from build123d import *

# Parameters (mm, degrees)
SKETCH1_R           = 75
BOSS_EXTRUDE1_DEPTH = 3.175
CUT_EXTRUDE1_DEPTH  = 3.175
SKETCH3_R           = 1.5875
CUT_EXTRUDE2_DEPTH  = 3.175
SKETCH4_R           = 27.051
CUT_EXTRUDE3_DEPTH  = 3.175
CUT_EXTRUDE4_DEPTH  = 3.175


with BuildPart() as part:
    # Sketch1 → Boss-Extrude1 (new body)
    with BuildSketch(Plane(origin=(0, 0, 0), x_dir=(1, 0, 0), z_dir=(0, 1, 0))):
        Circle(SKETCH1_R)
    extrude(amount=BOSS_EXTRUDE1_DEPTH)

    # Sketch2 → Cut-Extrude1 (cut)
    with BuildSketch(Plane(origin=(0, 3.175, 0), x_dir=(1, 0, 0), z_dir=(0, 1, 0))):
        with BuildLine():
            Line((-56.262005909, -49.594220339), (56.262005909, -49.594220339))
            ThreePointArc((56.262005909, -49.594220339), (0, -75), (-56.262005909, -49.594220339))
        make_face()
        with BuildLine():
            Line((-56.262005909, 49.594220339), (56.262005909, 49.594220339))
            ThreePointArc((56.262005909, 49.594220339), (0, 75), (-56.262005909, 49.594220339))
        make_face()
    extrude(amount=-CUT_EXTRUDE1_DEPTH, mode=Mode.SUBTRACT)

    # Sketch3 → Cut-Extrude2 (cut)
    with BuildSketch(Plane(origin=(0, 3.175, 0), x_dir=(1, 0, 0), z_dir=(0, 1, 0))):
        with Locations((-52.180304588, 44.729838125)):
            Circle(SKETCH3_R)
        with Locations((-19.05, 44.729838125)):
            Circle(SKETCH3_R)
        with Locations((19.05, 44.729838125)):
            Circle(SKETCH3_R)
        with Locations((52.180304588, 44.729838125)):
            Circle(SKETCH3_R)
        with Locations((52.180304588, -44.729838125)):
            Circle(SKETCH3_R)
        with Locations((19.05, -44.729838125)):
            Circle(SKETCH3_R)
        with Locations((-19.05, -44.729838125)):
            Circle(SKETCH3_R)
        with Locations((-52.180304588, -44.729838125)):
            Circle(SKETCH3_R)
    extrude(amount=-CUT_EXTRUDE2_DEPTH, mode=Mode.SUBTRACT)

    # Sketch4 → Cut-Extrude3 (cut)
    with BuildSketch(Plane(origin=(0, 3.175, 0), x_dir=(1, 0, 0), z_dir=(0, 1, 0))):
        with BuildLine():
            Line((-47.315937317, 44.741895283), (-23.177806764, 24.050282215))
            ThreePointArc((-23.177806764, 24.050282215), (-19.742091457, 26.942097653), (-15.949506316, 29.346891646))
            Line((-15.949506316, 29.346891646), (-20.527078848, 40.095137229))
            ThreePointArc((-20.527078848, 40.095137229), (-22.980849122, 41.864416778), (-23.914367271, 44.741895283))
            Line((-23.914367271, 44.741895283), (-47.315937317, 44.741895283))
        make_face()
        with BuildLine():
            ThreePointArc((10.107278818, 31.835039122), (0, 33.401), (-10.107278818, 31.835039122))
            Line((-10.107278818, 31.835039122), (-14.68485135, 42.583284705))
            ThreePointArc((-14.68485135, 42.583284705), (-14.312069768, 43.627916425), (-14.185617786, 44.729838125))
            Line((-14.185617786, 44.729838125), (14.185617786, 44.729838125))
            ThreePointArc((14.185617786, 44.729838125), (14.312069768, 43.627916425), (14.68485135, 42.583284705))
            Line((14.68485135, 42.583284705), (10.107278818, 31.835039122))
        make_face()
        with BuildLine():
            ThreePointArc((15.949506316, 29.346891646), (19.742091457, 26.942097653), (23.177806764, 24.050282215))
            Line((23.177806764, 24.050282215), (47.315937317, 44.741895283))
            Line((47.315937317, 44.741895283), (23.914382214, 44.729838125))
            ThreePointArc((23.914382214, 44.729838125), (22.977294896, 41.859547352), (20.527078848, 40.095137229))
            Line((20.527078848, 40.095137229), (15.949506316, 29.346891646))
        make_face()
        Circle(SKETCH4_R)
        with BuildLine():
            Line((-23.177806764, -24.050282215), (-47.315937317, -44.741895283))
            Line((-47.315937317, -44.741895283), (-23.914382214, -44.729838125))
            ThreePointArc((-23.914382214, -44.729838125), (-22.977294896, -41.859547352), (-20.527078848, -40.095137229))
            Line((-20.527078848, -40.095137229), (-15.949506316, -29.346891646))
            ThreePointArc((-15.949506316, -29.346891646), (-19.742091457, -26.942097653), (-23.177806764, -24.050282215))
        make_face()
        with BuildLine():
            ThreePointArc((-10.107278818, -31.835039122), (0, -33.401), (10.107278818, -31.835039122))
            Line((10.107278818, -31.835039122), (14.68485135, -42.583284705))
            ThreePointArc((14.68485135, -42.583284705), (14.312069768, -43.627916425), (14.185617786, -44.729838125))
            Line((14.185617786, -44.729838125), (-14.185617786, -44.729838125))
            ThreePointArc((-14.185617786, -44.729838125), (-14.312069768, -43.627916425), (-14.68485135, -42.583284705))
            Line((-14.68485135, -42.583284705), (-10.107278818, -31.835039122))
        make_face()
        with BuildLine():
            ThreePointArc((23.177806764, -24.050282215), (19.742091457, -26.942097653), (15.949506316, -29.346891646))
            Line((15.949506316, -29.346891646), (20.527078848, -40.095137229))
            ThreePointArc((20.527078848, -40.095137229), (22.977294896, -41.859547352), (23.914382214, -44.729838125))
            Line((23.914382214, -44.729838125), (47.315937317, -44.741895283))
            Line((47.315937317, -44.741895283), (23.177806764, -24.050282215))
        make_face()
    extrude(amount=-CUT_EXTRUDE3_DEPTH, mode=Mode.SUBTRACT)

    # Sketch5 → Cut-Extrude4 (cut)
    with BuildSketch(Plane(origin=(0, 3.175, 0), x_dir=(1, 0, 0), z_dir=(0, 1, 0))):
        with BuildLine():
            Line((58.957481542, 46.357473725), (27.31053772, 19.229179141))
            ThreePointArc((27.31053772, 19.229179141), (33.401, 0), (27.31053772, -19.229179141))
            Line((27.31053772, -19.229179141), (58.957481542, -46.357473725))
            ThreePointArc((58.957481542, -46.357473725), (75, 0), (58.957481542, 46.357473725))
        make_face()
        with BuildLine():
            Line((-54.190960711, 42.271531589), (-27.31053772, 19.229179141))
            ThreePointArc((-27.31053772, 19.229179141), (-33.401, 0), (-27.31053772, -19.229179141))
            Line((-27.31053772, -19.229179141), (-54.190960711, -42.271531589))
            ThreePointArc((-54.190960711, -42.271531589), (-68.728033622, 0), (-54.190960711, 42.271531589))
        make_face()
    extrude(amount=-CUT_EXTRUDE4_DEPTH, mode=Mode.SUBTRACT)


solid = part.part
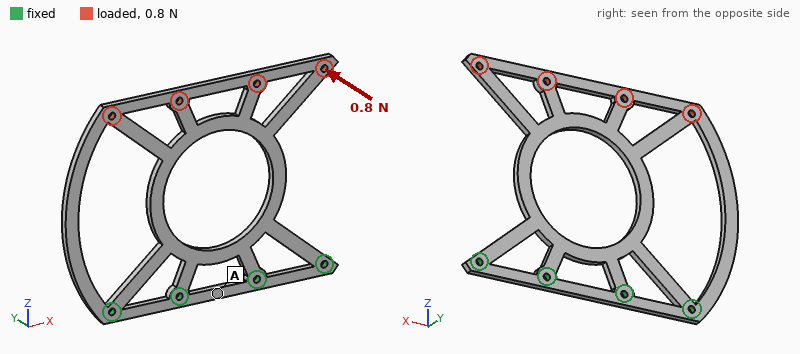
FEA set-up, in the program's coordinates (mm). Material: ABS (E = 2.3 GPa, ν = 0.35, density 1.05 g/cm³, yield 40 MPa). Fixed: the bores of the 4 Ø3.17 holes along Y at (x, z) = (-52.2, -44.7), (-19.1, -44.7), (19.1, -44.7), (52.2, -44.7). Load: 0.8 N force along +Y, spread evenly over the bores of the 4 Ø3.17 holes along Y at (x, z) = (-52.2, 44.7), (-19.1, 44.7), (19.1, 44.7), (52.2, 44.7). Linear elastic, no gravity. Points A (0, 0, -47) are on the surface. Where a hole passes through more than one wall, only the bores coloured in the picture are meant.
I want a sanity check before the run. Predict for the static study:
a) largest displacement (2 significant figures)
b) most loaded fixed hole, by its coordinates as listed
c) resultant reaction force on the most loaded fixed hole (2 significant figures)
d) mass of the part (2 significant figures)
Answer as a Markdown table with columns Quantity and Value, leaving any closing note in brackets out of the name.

| Quantity | Value |
|---|---|
| largest displacement | 1.8 mm |
| most loaded fixed hole, by its coordinates as listed | (19.1, -44.7) |
| resultant reaction force on the most loaded fixed hole | 0.30 N |
| mass of the part | 14 g |
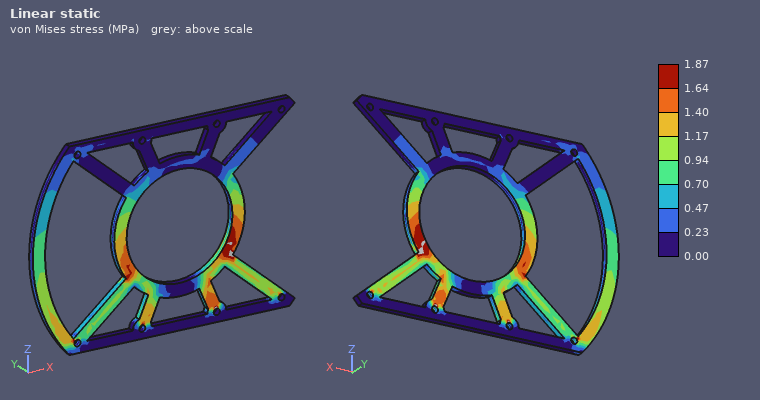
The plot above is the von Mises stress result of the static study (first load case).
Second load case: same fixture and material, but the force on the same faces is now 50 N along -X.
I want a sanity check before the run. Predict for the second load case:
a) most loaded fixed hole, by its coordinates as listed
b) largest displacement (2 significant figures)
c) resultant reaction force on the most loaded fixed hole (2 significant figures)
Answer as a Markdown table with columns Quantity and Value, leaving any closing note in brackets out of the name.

| Quantity | Value |
|---|---|
| most loaded fixed hole, by its coordinates as listed | (-52.2, -44.7) |
| largest displacement | 1.8 mm |
| resultant reaction force on the most loaded fixed hole | 66 N |
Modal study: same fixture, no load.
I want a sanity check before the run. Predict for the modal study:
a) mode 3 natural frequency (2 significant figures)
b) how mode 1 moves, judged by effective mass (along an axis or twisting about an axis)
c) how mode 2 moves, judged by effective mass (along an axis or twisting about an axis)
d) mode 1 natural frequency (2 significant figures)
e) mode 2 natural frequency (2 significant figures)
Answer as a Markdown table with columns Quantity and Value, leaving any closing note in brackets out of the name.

| Quantity | Value |
|---|---|
| mode 3 natural frequency | 290 Hz |
| how mode 1 moves, judged by effective mass | along Y |
| how mode 2 moves, judged by effective mass | twisting about Z |
| mode 1 natural frequency | 55 Hz |
| mode 2 natural frequency | 110 Hz |
